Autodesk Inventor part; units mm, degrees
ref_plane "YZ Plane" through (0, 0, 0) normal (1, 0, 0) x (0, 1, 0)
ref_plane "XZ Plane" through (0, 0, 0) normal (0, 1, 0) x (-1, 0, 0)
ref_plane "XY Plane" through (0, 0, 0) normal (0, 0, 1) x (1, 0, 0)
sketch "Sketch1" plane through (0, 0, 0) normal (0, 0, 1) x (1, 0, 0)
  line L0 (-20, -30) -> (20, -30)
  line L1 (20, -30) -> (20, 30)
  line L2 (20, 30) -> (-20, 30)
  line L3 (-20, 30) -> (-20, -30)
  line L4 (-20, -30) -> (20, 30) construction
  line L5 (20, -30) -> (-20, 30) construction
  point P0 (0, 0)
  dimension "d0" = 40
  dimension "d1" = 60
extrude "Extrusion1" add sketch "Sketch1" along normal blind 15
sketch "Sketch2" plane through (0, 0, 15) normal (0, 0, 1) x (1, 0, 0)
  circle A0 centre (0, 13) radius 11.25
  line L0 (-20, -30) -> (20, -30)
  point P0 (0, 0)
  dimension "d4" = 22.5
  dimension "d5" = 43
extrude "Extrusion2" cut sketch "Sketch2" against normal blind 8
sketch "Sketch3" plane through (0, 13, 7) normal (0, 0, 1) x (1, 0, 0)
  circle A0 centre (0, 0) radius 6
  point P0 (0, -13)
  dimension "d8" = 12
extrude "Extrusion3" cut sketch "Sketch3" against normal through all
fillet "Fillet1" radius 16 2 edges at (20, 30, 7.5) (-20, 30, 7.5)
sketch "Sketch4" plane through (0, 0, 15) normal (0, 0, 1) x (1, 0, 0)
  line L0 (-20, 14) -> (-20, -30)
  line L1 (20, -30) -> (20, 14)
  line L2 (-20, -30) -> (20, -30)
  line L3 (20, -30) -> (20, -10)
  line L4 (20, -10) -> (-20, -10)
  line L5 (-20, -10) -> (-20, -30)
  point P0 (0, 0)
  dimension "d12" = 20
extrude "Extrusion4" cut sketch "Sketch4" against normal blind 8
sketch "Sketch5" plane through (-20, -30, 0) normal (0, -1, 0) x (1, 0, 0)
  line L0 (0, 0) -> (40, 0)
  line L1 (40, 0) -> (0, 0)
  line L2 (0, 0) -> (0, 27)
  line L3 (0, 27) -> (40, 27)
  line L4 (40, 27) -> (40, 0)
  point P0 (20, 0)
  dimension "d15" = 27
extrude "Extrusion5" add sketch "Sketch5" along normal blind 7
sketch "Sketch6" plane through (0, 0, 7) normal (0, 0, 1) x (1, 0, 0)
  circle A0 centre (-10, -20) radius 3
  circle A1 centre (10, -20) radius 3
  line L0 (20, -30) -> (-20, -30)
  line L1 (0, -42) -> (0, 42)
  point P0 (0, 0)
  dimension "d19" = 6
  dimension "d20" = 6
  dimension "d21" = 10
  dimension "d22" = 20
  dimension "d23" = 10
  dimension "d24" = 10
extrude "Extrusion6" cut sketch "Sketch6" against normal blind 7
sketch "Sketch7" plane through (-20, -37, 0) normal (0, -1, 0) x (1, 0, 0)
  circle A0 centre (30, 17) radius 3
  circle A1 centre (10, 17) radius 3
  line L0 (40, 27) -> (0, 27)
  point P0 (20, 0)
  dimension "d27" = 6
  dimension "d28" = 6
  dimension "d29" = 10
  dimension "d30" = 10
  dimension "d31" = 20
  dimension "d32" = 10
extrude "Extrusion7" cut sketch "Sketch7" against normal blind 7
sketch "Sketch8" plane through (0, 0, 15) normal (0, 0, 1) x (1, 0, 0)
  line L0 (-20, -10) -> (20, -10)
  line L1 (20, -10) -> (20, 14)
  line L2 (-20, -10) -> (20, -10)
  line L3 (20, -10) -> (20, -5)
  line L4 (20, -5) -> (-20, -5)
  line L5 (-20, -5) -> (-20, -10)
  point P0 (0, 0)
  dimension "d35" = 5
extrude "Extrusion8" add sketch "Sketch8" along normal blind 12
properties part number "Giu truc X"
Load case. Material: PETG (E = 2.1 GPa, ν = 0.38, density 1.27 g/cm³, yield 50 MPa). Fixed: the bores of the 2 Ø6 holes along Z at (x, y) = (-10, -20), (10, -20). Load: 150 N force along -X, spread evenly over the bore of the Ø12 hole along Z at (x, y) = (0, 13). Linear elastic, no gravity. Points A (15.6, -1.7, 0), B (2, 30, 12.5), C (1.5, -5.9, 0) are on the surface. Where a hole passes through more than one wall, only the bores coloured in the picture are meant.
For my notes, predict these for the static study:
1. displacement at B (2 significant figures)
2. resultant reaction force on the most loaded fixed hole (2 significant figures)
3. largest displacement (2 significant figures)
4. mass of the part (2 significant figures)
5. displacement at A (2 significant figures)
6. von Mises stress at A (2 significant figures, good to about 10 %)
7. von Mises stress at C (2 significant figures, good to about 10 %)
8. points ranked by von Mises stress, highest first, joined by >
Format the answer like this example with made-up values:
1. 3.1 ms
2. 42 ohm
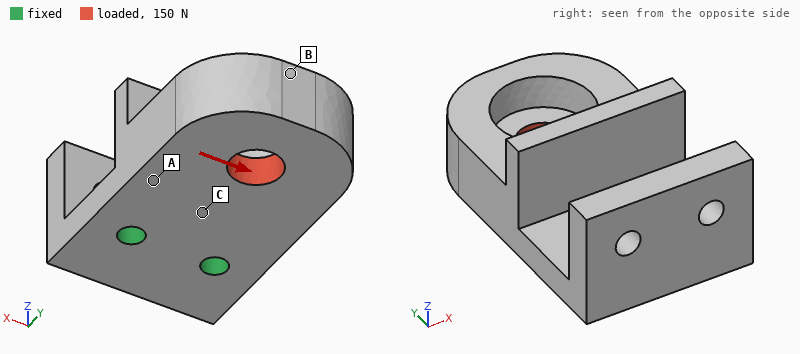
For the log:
1. 71 µm
2. 220 N
3. 84 µm
4. 42 g
5. 33 µm
6. 1.1 MPa
7. 1.9 MPa
8. C > A > B
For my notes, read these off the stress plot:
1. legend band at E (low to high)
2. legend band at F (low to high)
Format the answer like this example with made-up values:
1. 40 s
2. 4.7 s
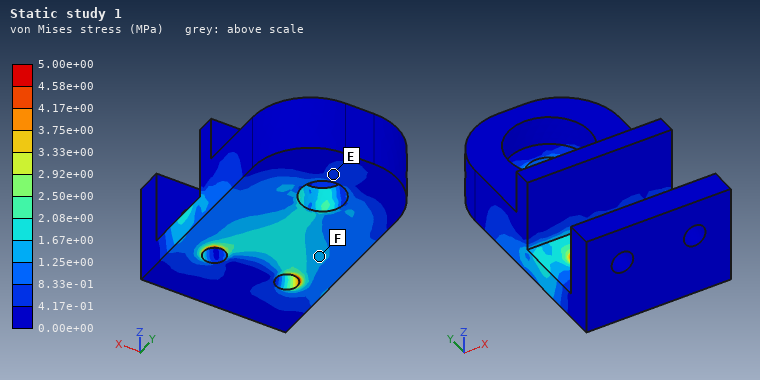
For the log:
1. 4.17e-01 to 8.33e-01 MPa
2. 1.25e+00 to 1.67e+00 MPa
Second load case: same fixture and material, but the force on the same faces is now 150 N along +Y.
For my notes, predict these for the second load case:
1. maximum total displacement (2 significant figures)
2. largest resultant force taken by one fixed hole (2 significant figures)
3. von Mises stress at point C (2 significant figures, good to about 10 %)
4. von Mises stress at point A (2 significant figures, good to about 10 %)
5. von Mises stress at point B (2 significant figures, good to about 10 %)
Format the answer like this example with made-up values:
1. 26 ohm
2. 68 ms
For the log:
1. 21 µm
2. 76 N
3. 0.66 MPa
4. 0.58 MPa
5. 0.26 MPa
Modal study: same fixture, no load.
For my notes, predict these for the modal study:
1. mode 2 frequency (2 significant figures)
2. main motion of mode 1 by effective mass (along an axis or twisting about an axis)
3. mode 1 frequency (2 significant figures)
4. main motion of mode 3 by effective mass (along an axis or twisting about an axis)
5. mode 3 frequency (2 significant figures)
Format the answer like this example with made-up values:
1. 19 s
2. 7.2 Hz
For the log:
1. 1500 Hz
2. along Z
3. 560 Hz
4. along X
5. 1700 Hz
